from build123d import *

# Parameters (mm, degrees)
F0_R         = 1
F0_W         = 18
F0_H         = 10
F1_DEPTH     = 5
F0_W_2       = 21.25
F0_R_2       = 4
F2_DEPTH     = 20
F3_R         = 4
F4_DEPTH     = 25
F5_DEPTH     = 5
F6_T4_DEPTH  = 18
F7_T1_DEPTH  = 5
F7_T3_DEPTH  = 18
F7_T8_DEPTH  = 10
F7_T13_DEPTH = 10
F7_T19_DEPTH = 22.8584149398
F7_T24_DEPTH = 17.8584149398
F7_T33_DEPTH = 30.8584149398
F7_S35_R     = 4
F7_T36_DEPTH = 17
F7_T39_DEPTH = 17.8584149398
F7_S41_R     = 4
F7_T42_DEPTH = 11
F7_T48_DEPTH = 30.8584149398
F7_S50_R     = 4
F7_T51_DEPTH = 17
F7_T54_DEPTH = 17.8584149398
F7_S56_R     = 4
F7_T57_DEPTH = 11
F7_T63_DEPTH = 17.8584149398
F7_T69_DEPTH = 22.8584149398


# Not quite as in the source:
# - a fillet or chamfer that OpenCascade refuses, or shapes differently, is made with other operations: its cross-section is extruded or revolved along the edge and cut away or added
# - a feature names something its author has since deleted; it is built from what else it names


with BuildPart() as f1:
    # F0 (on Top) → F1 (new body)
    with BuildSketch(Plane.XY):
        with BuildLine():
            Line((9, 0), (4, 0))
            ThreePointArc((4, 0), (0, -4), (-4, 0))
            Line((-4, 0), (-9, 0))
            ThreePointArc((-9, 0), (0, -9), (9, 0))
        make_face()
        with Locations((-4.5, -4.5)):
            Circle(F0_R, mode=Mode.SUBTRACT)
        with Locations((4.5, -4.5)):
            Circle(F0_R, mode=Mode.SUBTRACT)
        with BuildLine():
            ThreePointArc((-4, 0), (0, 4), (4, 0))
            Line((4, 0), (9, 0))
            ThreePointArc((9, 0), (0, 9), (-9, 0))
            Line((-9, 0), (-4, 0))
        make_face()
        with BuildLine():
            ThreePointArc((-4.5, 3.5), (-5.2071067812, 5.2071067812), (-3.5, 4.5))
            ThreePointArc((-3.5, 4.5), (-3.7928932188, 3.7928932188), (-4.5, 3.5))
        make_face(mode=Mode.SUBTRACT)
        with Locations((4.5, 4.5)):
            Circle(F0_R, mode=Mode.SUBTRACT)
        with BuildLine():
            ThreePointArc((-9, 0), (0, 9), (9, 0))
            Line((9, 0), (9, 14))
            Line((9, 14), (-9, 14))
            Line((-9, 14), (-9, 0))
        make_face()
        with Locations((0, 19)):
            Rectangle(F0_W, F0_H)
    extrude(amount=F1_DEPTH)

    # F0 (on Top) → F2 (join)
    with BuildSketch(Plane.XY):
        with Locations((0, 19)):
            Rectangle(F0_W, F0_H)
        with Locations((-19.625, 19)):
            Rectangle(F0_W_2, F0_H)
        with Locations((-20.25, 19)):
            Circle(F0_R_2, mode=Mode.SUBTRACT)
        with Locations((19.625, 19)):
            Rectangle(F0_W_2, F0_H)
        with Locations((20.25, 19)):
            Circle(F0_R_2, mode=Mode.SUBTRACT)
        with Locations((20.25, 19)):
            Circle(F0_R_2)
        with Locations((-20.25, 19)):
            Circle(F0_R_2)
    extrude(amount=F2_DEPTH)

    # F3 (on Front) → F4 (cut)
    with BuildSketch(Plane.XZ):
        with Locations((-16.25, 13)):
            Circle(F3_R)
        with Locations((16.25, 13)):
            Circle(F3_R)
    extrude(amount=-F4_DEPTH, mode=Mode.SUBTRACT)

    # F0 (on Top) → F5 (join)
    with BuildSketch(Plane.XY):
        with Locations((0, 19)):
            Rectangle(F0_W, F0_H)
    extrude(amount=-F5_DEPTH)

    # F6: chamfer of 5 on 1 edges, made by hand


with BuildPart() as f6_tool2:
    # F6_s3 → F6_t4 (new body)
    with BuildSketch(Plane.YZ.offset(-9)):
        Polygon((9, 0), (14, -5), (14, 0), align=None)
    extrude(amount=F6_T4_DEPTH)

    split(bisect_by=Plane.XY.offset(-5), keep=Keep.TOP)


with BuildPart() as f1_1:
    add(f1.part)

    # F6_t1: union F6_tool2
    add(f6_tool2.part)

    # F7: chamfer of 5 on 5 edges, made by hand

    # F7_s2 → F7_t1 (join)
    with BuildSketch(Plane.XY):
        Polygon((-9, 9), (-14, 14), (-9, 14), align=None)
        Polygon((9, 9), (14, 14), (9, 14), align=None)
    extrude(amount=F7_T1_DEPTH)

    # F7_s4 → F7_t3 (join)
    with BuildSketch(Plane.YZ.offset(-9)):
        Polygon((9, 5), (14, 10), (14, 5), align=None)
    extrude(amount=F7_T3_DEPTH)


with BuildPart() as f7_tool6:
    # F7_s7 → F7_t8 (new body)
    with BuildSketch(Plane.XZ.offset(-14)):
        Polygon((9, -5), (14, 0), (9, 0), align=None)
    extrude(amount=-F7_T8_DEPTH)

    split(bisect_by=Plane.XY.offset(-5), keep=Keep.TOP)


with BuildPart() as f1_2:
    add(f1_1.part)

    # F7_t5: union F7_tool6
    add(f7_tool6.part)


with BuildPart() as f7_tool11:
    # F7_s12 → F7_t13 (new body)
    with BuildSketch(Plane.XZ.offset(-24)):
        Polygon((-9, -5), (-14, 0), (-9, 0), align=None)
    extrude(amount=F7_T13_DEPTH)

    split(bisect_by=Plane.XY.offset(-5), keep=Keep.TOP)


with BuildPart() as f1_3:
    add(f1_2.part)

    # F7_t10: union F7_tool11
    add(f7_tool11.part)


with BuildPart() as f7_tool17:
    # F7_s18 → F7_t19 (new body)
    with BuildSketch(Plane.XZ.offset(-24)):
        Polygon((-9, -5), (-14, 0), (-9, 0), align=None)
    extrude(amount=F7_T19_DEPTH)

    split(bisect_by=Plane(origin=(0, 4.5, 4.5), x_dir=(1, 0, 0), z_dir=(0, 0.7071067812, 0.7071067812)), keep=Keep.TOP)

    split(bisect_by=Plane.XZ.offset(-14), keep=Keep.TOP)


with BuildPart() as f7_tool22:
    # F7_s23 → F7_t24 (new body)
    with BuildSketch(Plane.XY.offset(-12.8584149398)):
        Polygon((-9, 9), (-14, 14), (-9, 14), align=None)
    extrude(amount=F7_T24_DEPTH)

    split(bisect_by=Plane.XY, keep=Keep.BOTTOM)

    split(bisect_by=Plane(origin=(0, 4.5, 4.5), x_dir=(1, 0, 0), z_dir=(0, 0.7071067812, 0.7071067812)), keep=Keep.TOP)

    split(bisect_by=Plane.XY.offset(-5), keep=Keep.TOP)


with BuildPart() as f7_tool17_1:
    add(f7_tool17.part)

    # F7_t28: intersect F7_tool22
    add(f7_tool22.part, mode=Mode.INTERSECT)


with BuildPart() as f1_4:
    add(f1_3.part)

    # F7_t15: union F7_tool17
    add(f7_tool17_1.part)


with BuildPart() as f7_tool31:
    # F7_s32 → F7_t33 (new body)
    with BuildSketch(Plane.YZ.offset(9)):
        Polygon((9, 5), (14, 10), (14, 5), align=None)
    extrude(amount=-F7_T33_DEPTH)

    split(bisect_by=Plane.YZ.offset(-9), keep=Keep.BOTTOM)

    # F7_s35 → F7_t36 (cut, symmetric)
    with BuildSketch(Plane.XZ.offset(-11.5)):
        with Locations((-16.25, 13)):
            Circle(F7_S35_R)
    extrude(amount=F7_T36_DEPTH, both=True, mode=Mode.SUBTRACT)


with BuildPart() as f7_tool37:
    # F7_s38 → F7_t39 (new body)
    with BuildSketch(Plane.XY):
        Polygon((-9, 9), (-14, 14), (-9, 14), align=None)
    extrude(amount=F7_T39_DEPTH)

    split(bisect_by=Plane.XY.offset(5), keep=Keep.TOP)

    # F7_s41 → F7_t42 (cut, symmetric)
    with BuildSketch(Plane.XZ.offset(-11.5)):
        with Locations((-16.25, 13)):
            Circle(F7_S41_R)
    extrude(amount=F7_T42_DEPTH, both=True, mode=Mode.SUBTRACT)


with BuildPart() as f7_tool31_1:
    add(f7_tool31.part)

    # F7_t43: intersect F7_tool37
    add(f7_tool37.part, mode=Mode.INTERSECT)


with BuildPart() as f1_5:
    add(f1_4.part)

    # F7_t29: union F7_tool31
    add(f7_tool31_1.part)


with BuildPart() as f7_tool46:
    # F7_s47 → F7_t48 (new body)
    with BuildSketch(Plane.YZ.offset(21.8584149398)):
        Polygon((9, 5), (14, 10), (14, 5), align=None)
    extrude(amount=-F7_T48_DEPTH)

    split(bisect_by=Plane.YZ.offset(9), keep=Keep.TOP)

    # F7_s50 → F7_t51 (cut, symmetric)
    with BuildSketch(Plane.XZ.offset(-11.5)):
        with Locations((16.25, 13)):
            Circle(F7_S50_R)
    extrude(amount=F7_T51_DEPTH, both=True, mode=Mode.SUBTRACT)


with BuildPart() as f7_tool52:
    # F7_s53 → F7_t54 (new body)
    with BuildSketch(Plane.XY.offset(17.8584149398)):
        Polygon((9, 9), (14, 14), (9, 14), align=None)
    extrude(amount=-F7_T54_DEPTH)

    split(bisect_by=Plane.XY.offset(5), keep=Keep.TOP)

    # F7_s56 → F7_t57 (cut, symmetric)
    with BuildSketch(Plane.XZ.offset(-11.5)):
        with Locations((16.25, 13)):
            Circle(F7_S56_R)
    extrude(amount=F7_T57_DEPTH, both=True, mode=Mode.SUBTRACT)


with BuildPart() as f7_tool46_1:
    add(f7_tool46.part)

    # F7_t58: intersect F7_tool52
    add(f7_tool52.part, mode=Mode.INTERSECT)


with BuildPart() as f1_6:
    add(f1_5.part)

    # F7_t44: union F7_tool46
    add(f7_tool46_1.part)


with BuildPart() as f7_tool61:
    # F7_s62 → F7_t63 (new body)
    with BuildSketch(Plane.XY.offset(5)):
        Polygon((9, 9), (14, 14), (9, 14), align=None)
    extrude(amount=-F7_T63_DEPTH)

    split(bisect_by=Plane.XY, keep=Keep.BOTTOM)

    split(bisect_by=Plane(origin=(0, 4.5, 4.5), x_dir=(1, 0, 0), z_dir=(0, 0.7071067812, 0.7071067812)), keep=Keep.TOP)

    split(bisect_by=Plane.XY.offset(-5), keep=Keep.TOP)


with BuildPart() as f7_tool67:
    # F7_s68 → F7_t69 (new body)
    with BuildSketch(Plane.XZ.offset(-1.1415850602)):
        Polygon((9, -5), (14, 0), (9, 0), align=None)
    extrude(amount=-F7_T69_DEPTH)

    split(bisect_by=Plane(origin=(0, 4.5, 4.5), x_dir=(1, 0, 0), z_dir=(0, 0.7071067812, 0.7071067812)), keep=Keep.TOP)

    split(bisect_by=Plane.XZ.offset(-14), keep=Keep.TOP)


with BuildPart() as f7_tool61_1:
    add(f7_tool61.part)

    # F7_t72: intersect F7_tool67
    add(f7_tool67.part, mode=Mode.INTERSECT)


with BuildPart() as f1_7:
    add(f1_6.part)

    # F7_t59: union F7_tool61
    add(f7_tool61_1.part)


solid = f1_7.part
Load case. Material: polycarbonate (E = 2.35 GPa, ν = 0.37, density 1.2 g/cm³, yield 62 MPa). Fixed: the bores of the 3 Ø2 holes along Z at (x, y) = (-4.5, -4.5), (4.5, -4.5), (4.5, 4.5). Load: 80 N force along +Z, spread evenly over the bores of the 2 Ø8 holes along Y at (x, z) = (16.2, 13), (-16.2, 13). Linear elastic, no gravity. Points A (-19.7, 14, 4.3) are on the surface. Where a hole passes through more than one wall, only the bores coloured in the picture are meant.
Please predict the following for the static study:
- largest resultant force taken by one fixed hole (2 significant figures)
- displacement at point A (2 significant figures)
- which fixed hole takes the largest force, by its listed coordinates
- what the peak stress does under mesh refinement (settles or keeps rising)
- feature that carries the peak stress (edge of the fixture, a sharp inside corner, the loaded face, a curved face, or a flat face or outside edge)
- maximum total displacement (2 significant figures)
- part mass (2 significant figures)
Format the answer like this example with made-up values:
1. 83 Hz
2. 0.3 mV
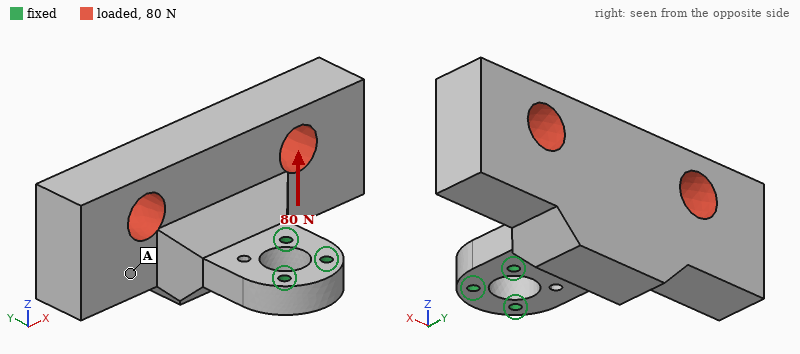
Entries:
1. 100 N
2. 0.34 mm
3. (4.5, 4.5)
4. keeps rising
5. edge of the fixture
6. 0.73 mm
7. 17 g
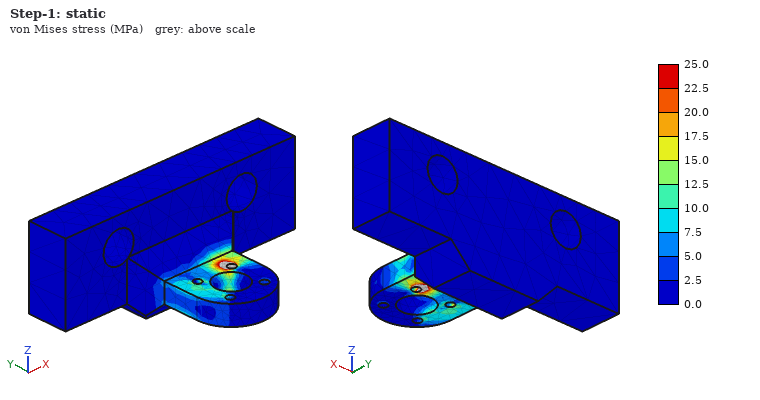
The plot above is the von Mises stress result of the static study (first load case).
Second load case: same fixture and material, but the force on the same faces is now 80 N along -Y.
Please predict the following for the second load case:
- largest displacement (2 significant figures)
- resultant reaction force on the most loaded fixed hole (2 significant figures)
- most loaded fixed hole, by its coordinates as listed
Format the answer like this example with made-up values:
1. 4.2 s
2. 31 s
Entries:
1. 0.53 mm
2. 57 N
3. (4.5, 4.5)
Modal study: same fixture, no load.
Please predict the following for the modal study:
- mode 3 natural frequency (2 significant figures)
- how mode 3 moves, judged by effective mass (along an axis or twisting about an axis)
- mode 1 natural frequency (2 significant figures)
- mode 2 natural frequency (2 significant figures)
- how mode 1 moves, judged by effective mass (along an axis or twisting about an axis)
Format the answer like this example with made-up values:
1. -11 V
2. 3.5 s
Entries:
1. 1100 Hz
2. along X
3. 490 Hz
4. 700 Hz
5. along Z
